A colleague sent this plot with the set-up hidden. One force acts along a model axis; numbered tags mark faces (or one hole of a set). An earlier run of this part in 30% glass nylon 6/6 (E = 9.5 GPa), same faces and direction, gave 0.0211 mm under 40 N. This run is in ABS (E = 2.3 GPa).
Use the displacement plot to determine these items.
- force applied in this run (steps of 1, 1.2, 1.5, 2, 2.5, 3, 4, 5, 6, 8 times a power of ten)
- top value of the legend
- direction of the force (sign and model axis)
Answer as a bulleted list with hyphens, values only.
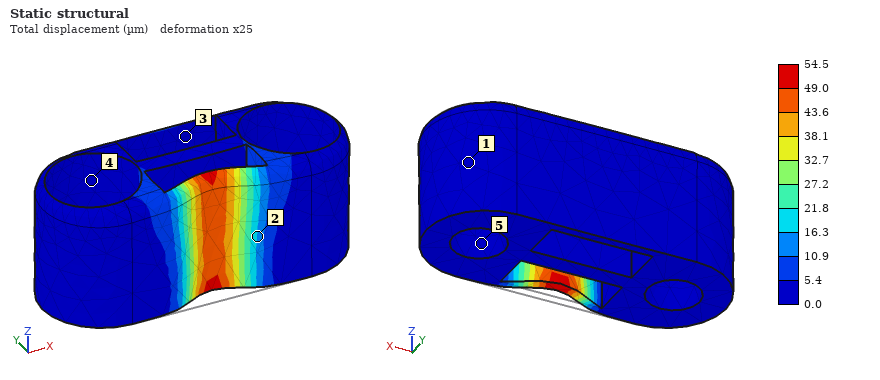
- 25 N
- 54.5 µm
- +Y
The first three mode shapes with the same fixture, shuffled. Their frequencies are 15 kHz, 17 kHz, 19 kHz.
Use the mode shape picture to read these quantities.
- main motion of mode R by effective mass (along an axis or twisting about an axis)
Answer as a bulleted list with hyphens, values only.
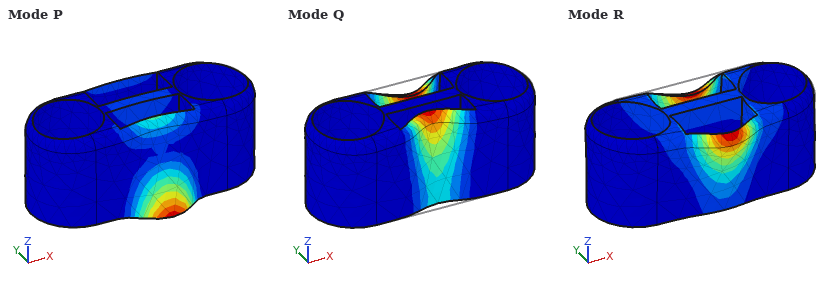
- along Y
